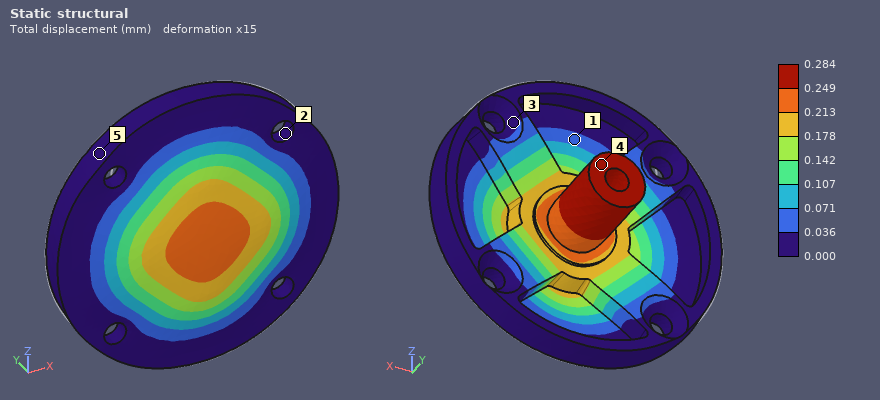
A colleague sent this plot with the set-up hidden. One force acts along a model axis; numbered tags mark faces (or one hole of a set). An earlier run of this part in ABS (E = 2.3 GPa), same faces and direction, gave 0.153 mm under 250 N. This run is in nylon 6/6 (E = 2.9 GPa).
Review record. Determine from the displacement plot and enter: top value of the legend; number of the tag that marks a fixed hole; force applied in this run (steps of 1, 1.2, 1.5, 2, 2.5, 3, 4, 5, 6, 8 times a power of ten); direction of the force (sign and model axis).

0.284 mm
2
600 N
-Y
